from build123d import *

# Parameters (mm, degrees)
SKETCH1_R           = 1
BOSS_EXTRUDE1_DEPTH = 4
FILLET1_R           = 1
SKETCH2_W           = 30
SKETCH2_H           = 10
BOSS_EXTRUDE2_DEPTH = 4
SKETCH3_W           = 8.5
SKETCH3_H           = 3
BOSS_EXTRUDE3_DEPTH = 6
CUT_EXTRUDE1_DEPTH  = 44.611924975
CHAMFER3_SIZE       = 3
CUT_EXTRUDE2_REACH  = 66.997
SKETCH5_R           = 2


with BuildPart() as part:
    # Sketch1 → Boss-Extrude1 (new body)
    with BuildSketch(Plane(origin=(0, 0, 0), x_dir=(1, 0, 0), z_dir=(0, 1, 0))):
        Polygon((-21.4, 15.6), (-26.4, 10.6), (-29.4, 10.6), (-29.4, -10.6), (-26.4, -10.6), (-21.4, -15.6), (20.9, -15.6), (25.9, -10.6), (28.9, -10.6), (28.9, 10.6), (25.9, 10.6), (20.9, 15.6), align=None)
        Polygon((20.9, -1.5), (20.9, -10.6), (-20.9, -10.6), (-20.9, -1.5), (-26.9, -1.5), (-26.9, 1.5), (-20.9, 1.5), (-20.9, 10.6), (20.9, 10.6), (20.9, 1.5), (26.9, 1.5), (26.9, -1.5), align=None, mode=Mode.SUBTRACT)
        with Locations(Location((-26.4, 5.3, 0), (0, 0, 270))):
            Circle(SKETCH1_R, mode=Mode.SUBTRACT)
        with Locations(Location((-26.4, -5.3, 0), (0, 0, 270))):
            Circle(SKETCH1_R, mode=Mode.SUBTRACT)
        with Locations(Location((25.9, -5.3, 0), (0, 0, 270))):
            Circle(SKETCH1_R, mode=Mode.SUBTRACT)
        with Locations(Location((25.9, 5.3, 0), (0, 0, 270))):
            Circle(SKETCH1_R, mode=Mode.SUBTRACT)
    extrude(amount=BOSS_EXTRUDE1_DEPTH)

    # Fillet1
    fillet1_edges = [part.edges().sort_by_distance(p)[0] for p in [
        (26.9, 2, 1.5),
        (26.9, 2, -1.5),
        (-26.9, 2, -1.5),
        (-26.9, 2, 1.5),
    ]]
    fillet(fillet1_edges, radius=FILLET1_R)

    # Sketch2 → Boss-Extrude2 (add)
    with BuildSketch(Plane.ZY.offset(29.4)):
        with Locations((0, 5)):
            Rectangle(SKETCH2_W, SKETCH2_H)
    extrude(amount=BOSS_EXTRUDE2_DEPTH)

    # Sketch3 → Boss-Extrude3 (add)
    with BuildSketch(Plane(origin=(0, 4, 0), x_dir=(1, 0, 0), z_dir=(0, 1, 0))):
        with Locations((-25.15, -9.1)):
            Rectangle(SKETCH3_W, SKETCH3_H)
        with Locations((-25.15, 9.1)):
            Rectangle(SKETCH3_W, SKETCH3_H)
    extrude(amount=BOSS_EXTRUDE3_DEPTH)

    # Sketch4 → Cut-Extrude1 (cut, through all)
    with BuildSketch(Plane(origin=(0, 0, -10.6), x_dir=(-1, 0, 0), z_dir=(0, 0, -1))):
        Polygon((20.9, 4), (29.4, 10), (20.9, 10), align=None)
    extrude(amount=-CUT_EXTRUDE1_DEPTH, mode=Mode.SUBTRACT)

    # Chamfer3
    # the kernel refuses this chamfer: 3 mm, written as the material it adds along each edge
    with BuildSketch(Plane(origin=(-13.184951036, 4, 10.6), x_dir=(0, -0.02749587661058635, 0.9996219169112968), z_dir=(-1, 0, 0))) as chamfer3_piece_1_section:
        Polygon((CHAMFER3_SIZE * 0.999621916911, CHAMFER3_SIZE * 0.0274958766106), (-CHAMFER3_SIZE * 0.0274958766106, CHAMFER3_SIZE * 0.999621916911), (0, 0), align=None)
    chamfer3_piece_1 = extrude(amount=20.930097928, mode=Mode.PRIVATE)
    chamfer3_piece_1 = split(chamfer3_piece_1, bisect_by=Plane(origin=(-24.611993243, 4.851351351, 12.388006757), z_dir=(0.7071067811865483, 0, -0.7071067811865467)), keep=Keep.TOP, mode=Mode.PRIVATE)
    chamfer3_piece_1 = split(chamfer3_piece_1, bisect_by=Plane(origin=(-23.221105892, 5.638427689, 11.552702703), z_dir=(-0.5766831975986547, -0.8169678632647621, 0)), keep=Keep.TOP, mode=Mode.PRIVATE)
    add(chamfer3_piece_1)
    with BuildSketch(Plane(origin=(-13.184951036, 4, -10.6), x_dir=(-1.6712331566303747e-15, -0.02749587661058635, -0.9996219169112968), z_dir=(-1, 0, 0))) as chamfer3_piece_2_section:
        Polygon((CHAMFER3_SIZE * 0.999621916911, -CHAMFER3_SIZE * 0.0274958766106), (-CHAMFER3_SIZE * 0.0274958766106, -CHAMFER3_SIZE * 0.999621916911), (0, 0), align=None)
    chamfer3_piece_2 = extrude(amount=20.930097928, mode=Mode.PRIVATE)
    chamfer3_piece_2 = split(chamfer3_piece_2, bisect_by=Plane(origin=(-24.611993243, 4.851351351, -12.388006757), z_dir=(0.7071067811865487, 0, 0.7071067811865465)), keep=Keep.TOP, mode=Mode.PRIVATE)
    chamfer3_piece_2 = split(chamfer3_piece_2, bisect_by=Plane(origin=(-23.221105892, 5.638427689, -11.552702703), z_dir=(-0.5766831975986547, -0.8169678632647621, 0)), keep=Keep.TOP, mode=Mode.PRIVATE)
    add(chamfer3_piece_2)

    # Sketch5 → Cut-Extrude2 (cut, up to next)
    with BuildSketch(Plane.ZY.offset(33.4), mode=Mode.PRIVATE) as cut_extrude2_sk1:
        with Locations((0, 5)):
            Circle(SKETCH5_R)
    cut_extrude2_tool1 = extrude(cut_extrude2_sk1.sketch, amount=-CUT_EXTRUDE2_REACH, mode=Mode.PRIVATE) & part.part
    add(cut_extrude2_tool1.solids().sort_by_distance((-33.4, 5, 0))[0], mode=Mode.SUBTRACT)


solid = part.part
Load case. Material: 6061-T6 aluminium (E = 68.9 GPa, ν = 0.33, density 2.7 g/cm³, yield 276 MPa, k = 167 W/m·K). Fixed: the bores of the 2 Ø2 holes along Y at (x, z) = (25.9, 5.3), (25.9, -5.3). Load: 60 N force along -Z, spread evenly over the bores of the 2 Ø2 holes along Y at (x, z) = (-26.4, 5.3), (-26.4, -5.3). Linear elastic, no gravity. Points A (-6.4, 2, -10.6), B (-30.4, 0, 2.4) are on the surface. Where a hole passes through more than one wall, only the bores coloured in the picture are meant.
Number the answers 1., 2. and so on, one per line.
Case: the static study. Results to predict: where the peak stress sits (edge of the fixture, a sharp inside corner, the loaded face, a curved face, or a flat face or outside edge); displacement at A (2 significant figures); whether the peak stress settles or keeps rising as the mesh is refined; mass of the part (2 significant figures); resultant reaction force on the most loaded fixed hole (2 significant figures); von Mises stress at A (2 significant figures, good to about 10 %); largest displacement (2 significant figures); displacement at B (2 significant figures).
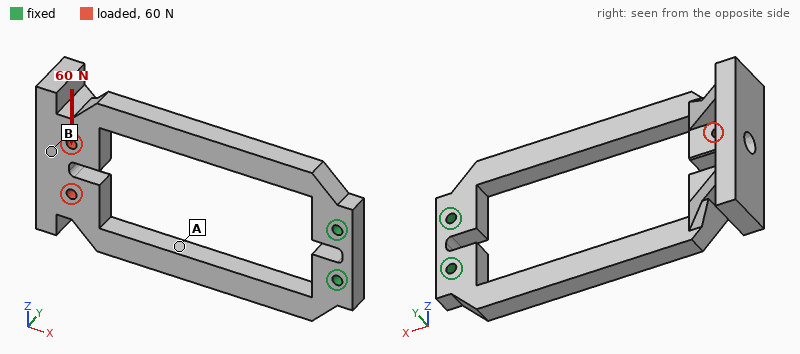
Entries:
1. edge of the fixture
2. 0.14 mm
3. keeps rising
4. 12 g
5. 140 N
6. 18 MPa
7. 0.21 mm
8. 0.21 mm
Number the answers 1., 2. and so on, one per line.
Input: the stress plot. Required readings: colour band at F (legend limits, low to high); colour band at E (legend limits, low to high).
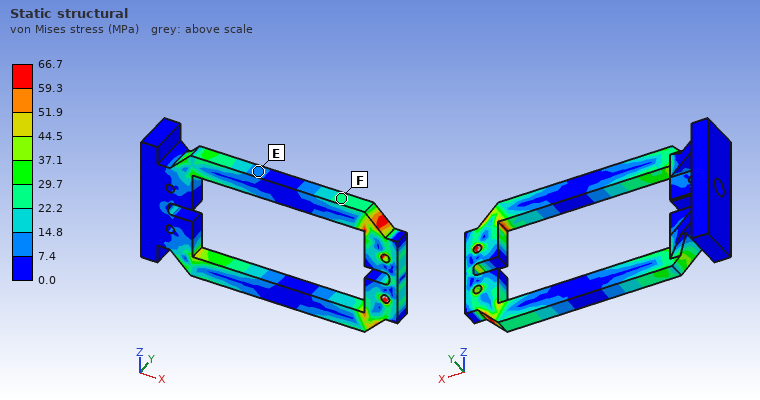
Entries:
1. 22.2 to 29.7 MPa
2. 7.4 to 14.8 MPa
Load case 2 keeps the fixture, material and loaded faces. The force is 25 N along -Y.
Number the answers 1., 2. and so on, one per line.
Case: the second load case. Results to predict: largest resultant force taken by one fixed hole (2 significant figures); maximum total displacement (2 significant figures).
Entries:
1. 13 N
2. 0.48 mm
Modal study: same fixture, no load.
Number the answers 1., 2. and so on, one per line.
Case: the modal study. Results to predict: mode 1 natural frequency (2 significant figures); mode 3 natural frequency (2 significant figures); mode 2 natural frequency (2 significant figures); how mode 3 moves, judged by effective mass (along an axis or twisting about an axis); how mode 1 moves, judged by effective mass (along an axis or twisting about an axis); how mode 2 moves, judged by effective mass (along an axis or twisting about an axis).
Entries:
1. 470 Hz
2. 1800 Hz
3. 1000 Hz
4. twisting about X
5. along Y
6. along Z
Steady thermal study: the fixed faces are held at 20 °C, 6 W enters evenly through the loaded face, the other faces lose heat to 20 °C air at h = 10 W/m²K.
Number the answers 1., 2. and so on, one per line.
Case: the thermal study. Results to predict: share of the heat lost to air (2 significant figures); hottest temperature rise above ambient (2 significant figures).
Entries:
1. 17 %
2. 44 K
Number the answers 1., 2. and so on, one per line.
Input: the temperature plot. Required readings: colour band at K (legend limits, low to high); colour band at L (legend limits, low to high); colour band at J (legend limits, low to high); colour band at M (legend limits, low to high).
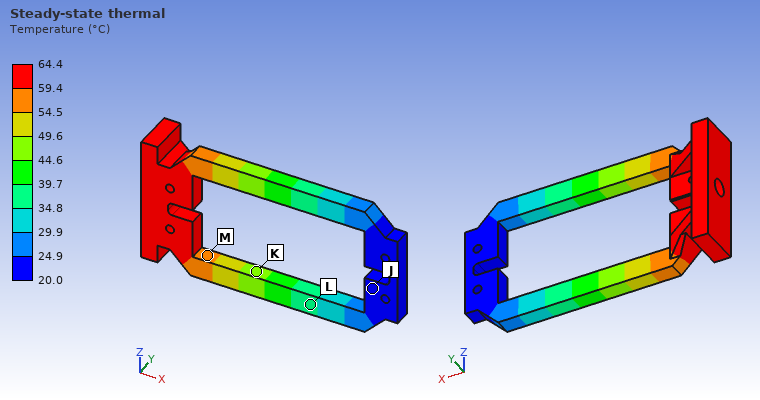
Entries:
1. 44.6 to 49.6 °C
2. 34.8 to 39.7 °C
3. 20.0 to 24.9 °C
4. 54.5 to 59.4 °C
